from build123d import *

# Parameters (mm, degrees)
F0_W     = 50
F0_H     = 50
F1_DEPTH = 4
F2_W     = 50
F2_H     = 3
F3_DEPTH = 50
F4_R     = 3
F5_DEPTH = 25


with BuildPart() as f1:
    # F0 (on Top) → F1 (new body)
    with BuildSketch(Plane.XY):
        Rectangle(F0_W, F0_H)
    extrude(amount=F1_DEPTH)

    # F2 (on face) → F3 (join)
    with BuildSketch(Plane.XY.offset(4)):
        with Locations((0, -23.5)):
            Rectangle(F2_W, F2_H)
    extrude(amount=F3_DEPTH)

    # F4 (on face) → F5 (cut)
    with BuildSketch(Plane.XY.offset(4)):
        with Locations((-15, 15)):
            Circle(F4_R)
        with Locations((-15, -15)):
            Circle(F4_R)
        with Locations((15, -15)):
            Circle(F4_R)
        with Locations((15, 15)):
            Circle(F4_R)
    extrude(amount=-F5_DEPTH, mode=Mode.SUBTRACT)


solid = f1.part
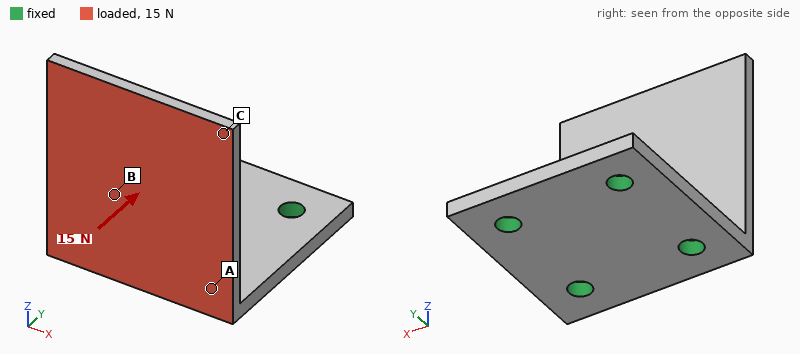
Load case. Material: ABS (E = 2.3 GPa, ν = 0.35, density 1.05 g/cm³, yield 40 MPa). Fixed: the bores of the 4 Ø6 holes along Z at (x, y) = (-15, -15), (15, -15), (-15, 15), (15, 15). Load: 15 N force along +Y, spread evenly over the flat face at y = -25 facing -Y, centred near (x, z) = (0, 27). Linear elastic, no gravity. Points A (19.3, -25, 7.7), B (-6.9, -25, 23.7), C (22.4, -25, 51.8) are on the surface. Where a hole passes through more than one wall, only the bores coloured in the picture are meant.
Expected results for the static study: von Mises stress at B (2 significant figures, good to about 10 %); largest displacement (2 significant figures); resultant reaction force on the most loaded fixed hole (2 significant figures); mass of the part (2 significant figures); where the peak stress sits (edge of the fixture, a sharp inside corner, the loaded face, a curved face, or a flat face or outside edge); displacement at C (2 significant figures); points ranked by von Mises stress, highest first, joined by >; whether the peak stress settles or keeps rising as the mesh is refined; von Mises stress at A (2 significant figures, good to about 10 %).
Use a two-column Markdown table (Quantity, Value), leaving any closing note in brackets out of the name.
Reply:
| Quantity | Value |
|---|---|
| von Mises stress at B | 1.5 MPa |
| largest displacement | 1.1 mm |
| resultant reaction force on the most loaded fixed hole | 6.7 N |
| mass of the part | 18 g |
| where the peak stress sits | edge of the fixture |
| displacement at C | 1.00 mm |
| points ranked by von Mises stress, highest first, joined by > | A > B > C |
| whether the peak stress settles or keeps rising as the mesh is refined | keeps rising |
| von Mises stress at A | 3.5 MPa |
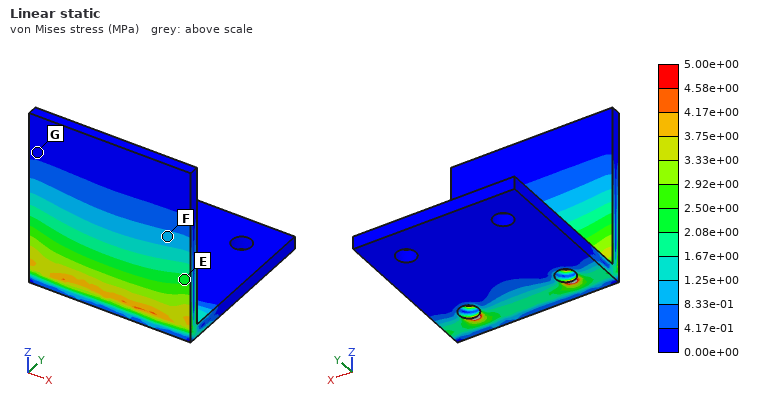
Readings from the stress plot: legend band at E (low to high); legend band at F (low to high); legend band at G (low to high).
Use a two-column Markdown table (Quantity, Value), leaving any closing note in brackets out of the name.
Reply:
| Quantity | Value |
|---|---|
| legend band at E | 2.08e+00 to 2.50e+00 MPa |
| legend band at F | 8.33e-01 to 1.25e+00 MPa |
| legend band at G | 0.00e+00 to 4.17e-01 MPa |
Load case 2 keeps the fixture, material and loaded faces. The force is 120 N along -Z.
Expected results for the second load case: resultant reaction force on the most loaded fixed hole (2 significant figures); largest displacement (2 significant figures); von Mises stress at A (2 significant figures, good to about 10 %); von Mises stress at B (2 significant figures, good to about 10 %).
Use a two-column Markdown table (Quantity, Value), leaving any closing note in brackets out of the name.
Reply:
| Quantity | Value |
|---|---|
| resultant reaction force on the most loaded fixed hole | 63 N |
| largest displacement | 0.94 mm |
| von Mises stress at A | 2.6 MPa |
| von Mises stress at B | 1.6 MPa |
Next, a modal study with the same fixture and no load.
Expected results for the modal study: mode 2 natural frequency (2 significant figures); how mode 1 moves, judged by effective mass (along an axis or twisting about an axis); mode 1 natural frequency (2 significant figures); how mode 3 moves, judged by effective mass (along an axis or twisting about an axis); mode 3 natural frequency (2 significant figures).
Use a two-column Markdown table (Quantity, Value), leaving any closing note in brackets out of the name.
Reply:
| Quantity | Value |
|---|---|
| mode 2 natural frequency | 640 Hz |
| how mode 1 moves, judged by effective mass | along Y |
| mode 1 natural frequency | 250 Hz |
| how mode 3 moves, judged by effective mass | along X |
| mode 3 natural frequency | 1500 Hz |
